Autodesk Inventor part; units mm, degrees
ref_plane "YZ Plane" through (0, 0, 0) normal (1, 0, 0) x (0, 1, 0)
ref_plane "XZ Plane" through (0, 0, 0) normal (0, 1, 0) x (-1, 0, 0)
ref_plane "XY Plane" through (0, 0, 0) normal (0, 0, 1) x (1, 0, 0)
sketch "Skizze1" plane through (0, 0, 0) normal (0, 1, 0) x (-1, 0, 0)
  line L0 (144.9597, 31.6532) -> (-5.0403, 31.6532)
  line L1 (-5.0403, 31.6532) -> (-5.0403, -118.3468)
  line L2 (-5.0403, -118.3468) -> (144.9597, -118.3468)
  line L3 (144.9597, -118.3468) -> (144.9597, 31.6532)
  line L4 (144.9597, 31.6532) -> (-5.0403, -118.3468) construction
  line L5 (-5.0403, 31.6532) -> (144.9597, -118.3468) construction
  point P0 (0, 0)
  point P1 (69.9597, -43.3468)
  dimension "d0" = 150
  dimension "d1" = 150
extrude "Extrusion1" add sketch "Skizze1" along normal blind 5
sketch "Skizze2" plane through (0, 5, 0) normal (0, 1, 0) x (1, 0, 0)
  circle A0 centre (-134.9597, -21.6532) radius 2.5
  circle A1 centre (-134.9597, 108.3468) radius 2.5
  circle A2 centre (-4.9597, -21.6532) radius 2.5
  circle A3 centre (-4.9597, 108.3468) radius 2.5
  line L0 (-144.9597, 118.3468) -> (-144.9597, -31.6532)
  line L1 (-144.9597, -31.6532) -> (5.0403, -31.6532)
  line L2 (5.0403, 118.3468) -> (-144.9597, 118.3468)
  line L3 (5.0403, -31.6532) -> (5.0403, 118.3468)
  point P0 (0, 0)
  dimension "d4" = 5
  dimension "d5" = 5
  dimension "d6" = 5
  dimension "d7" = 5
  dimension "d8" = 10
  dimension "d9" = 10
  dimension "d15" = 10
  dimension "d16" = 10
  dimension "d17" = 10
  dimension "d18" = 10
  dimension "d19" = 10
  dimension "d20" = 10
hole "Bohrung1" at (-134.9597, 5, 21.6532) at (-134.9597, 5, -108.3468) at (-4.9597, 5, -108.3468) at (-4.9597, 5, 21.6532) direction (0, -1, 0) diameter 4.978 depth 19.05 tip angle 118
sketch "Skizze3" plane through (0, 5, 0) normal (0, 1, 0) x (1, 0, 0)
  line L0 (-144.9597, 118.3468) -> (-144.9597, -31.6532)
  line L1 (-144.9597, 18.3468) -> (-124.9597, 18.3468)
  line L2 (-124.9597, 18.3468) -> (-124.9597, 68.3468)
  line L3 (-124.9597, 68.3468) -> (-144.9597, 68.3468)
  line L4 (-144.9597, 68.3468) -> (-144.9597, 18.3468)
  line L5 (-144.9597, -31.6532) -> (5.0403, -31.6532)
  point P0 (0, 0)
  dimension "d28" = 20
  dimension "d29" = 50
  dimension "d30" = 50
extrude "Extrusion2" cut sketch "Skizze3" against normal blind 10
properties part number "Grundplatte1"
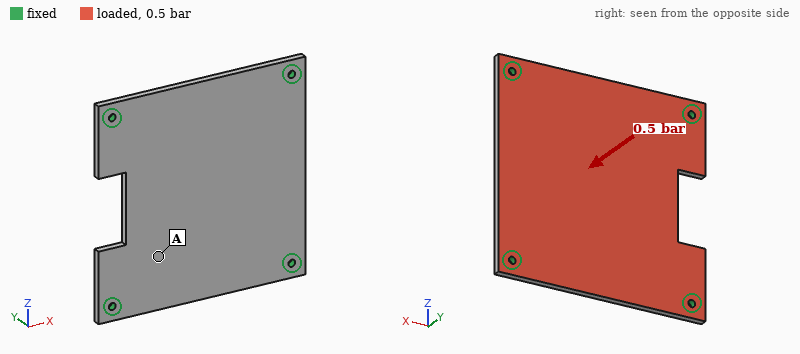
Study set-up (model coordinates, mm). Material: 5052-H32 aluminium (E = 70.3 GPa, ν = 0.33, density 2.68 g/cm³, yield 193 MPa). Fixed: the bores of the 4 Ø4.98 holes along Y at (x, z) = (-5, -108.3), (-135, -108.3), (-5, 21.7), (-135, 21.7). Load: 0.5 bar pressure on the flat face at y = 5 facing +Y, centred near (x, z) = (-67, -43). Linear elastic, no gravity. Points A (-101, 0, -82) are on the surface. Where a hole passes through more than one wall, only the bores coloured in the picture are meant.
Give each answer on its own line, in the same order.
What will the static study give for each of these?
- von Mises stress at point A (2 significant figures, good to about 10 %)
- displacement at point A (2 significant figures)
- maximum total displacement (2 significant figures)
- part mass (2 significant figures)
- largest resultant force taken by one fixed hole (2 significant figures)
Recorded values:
7.1 MPa
0.094 mm
0.15 mm
290 g
280 N
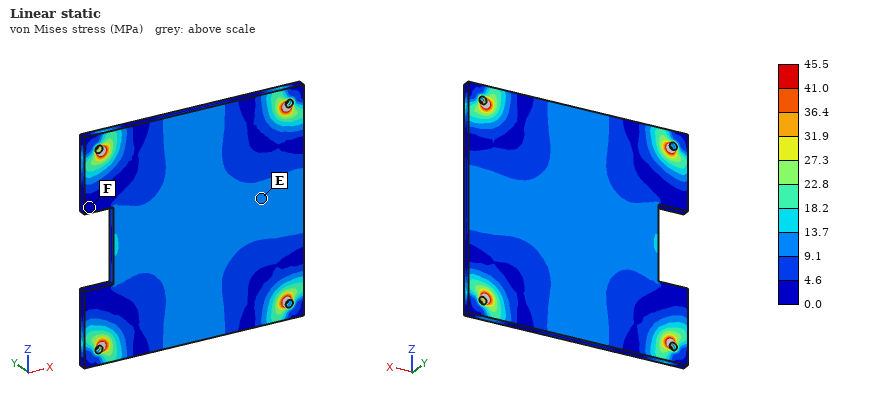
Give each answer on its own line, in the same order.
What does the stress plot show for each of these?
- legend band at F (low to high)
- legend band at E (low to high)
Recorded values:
0.0 to 4.6 MPa
9.1 to 13.7 MPa
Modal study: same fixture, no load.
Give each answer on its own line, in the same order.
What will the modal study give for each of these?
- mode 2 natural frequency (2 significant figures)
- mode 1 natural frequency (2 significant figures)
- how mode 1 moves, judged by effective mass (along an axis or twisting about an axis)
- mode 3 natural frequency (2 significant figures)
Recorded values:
1700 Hz
960 Hz
along Y
1700 Hz
